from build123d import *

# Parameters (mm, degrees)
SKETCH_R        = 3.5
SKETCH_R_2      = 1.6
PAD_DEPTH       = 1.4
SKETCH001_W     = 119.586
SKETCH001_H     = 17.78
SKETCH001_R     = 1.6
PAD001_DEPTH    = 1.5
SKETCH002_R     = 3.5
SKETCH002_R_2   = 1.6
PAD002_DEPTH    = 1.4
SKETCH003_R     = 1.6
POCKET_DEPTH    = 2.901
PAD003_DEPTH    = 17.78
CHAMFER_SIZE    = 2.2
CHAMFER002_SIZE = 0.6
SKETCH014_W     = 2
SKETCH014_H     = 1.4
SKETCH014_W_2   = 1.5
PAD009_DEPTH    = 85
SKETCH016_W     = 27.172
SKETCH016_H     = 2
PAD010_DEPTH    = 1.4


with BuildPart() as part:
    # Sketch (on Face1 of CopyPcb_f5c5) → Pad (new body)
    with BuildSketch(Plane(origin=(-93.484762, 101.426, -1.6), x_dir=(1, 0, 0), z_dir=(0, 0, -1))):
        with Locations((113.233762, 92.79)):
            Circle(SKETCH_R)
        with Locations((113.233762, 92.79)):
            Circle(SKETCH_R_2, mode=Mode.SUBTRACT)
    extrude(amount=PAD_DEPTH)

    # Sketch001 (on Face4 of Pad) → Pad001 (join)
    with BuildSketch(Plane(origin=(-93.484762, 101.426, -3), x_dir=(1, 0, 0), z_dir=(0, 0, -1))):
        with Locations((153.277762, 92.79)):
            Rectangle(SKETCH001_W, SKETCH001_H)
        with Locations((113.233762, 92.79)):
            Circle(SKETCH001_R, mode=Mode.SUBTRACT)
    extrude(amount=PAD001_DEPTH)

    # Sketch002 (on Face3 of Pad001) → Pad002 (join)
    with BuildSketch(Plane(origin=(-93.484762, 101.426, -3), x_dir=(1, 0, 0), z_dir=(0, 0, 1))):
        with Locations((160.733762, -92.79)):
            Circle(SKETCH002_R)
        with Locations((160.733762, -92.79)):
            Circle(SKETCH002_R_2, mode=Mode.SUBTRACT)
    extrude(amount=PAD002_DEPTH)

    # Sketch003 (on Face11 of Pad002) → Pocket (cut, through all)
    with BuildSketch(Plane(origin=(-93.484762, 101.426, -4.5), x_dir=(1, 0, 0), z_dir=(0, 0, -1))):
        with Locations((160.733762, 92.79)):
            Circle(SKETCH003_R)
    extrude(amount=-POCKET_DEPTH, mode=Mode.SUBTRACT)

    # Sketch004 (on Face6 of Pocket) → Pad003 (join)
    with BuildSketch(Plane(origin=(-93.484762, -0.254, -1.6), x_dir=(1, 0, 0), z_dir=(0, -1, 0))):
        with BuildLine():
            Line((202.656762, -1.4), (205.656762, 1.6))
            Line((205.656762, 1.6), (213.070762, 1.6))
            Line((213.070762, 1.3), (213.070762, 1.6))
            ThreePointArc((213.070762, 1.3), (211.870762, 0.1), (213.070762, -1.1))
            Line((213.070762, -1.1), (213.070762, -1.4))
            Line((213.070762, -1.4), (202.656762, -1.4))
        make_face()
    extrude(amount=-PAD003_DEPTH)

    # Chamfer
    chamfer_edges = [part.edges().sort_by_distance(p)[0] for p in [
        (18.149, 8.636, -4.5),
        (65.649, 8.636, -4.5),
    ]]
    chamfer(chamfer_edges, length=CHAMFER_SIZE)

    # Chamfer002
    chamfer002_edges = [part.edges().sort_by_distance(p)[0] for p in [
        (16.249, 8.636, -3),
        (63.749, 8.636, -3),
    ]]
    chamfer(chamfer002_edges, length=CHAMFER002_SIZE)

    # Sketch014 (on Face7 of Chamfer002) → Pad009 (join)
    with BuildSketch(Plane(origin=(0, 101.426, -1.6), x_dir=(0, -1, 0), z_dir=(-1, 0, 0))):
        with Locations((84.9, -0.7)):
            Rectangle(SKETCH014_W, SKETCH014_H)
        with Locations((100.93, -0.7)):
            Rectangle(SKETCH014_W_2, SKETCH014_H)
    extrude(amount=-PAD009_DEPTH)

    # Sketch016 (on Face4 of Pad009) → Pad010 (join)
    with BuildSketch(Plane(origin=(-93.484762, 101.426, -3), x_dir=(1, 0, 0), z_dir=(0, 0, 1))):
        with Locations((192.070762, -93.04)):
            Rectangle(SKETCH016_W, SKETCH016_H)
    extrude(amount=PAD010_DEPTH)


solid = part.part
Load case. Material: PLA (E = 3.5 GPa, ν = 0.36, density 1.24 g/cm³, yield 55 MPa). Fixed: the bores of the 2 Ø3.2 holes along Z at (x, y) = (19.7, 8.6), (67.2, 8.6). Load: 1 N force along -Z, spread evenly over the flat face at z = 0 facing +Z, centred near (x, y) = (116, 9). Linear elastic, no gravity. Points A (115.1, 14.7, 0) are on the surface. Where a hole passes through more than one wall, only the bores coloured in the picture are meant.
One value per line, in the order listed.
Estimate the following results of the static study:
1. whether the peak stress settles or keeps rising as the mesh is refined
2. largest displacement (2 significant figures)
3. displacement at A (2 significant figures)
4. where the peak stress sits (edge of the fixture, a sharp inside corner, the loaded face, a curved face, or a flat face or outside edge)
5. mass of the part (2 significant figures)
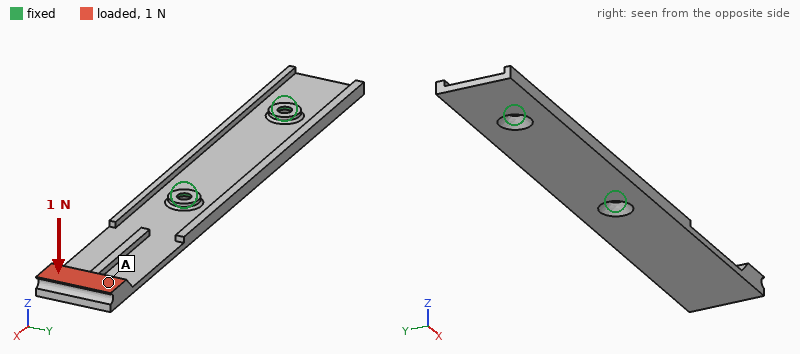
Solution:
keeps rising
1.2 mm
1.1 mm
edge of the fixture
5.1 g
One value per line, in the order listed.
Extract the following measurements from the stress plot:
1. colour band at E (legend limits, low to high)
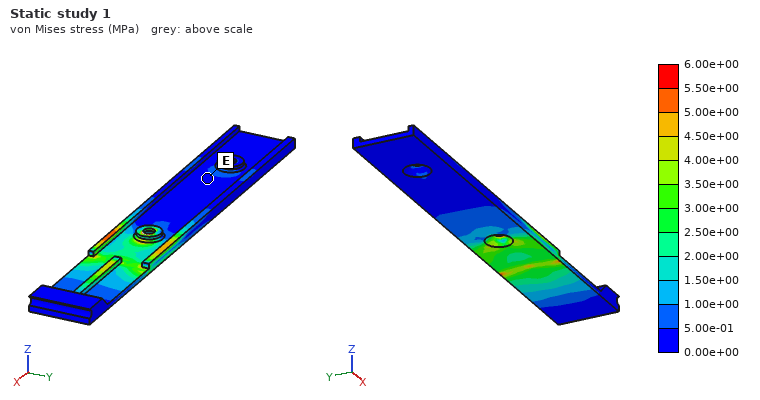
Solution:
0.00e+00 to 5.00e-01 MPa
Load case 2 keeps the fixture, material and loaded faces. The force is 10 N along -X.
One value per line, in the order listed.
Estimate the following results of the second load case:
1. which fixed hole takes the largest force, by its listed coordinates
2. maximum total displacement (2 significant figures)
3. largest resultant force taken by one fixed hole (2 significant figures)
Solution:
(67.2, 8.6)
1.3 mm
11 N
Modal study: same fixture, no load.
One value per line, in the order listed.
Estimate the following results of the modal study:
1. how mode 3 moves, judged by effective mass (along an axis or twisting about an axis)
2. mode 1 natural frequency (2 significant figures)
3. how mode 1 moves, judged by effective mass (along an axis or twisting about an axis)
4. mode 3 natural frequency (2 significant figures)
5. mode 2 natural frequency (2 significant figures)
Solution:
along Y
150 Hz
along Z
950 Hz
690 Hz
